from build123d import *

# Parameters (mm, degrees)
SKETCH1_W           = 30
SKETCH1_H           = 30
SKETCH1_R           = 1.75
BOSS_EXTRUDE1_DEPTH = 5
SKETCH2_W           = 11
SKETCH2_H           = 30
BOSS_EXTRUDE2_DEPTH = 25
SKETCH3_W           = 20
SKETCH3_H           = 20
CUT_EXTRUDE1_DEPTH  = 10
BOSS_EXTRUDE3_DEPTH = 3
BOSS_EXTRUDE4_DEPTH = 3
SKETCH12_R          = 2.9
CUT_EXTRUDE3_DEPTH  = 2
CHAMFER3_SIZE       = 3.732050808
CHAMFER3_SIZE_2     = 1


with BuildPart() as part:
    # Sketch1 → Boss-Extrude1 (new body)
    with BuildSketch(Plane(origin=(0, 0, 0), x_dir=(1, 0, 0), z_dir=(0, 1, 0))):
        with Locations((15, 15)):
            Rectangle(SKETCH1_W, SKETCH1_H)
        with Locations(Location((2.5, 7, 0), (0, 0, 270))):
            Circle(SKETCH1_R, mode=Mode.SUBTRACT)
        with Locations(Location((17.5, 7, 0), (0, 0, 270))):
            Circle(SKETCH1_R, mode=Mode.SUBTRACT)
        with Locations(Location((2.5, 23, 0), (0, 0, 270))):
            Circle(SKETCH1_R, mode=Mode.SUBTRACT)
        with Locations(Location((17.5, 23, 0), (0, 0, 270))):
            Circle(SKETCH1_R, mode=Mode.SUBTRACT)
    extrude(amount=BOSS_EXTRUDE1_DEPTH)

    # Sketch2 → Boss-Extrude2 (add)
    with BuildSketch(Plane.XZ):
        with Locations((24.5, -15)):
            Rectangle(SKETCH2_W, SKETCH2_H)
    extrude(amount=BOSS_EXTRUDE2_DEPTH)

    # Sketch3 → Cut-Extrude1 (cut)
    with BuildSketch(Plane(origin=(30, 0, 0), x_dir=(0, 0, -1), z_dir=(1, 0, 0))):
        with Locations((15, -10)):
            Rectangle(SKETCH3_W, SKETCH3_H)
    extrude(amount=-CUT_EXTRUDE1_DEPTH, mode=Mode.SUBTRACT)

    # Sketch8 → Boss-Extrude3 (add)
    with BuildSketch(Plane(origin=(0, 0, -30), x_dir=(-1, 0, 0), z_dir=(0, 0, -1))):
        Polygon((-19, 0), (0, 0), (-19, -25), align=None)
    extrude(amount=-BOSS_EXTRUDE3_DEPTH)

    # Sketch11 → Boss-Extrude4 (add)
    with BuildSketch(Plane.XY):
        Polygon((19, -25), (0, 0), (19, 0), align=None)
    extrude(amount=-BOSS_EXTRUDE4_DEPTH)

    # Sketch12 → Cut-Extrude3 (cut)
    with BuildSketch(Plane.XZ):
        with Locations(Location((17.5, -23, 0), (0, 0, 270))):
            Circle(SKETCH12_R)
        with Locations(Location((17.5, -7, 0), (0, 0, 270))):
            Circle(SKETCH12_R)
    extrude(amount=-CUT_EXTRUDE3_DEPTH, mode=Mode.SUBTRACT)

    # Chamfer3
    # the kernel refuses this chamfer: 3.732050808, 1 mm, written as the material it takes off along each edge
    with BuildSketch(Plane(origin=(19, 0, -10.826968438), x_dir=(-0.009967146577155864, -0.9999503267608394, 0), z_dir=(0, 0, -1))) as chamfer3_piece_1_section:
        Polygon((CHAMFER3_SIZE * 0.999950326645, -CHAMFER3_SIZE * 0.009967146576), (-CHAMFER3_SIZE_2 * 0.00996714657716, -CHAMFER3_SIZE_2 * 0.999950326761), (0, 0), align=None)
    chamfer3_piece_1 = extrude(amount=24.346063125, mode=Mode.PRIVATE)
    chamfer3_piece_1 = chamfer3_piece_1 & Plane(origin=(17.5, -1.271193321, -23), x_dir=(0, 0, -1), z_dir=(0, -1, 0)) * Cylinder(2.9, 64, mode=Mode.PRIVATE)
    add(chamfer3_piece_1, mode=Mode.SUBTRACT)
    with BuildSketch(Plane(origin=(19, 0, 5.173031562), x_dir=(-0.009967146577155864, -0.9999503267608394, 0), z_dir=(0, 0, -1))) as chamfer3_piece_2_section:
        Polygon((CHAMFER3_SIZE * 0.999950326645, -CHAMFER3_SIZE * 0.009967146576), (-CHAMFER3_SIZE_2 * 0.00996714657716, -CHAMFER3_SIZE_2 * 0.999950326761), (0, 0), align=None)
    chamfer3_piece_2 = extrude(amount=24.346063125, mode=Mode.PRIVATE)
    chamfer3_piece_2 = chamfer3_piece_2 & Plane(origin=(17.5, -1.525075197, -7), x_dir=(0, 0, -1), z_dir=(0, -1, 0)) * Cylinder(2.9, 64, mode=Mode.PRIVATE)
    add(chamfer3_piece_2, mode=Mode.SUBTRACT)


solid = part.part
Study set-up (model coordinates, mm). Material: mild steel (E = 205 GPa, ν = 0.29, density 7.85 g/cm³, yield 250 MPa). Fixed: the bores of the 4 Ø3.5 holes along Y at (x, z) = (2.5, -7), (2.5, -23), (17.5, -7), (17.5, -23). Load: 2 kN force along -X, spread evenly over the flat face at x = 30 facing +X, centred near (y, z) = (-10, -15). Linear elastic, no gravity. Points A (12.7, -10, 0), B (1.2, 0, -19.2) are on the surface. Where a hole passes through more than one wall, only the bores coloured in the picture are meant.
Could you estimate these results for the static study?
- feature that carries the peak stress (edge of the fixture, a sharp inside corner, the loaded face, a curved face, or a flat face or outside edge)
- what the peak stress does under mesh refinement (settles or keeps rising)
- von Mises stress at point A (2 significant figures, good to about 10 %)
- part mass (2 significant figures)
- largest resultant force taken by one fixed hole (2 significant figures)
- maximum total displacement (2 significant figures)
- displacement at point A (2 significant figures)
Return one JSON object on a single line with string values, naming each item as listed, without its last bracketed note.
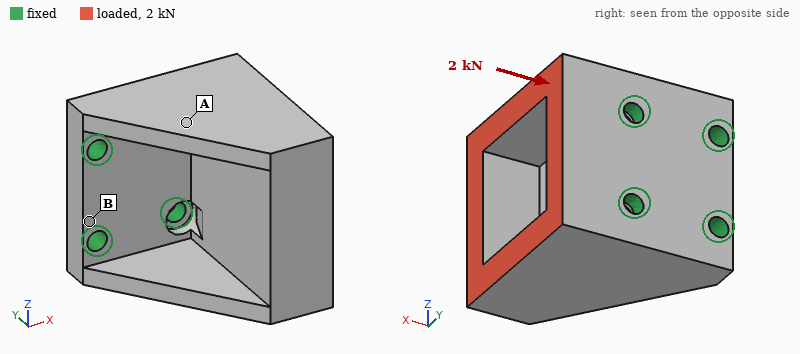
{"feature that carries the peak stress": "edge of the fixture", "what the peak stress does under mesh refinement": "keeps rising", "von Mises stress at point A": "25 MPa", "part mass": "78 g", "largest resultant force taken by one fixed hole": "1.0 kN", "maximum total displacement": "18 µm", "displacement at point A": "5.9 µm"}
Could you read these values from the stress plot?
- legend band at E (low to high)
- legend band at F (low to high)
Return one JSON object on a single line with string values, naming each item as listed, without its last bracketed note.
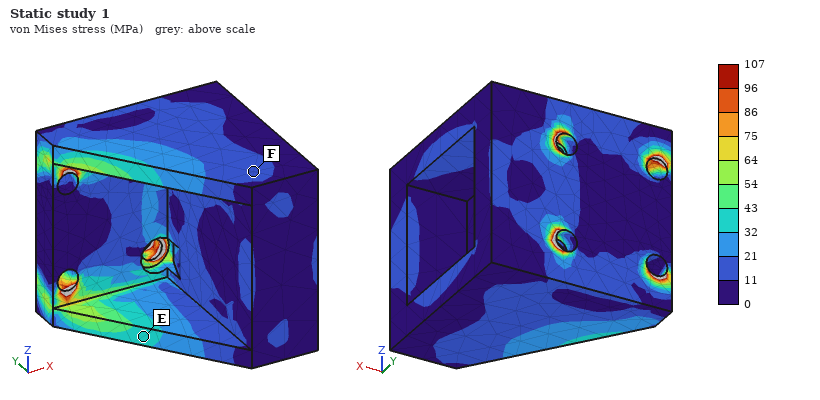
{"legend band at E": "32 to 43 MPa", "legend band at F": "11 to 21 MPa"}
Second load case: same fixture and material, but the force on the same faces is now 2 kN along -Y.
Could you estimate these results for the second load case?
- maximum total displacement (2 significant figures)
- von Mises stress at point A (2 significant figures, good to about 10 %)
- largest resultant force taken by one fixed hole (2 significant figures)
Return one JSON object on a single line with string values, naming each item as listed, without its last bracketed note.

{"maximum total displacement": "22 µm", "von Mises stress at point A": "20 MPa", "largest resultant force taken by one fixed hole": "1.7 kN"}
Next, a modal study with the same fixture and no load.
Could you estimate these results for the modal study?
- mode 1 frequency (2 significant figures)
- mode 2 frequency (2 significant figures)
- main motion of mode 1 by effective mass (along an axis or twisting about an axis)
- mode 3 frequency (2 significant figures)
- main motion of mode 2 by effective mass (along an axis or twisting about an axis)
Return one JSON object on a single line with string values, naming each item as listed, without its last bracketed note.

{"mode 1 frequency": "7800 Hz", "mode 2 frequency": "8200 Hz", "main motion of mode 1 by effective mass": "along Z", "mode 3 frequency": "13 kHz", "main motion of mode 2 by effective mass": "along X"}
